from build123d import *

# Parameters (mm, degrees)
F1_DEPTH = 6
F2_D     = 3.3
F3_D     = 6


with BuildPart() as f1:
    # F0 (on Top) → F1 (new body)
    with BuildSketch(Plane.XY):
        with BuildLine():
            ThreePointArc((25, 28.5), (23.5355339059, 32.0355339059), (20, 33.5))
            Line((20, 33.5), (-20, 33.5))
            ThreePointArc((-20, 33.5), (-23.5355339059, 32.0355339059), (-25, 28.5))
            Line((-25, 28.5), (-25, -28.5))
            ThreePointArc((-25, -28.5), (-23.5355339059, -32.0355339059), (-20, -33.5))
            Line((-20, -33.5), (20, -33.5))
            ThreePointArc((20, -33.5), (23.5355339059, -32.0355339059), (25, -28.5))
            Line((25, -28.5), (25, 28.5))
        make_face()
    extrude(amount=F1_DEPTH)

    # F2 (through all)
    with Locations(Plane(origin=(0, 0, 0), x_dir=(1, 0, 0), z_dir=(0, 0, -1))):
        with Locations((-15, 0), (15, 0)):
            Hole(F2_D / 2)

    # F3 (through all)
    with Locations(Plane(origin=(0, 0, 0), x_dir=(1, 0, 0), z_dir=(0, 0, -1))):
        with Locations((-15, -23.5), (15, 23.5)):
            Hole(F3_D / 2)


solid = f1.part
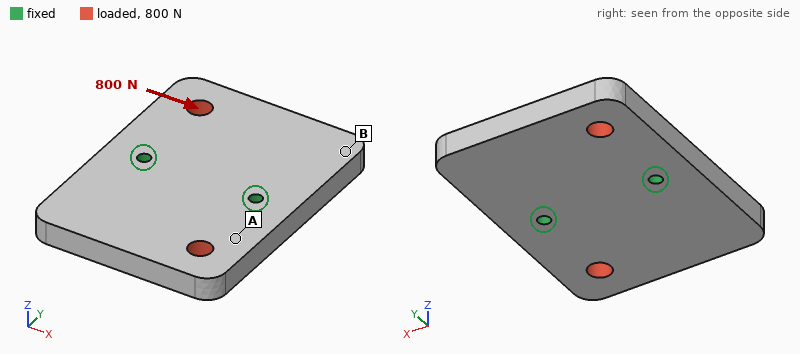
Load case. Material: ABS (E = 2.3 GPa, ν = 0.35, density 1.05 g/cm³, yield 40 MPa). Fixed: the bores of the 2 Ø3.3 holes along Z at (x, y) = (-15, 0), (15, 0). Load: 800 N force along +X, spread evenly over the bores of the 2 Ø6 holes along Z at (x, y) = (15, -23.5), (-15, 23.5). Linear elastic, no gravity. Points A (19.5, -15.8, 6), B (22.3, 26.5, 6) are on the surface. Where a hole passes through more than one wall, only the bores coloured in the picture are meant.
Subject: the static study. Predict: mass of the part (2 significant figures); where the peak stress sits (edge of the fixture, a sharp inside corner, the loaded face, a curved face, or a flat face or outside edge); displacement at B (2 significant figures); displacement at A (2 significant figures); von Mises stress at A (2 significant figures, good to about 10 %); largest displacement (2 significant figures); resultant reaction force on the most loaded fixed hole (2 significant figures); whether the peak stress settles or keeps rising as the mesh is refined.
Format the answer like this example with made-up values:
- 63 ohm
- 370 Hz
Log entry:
- 21 g
- edge of the fixture
- 55 µm
- 51 µm
- 2.5 MPa
- 87 µm
- 400 N
- keeps rising
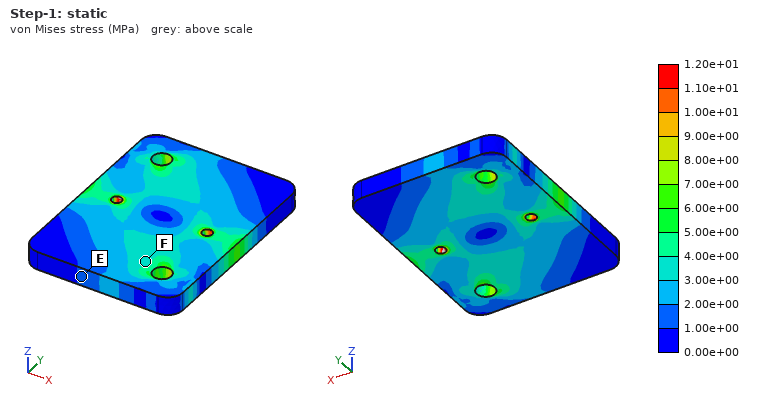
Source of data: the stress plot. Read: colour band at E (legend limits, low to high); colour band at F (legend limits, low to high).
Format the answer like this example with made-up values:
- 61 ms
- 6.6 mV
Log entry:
- 1.00e+00 to 2.00e+00 MPa
- 3.00e+00 to 4.00e+00 MPa
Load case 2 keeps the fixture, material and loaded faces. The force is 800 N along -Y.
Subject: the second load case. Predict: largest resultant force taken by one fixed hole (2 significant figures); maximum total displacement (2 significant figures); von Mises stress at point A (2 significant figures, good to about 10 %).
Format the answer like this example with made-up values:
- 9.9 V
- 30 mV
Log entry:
- 400 N
- 56 µm
- 3.8 MPa
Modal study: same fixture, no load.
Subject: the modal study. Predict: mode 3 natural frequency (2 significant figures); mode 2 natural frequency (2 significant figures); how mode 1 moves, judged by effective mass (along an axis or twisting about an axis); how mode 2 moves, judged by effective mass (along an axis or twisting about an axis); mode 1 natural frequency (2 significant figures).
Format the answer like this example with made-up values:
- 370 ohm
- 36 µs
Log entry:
- 2000 Hz
- 1300 Hz
- twisting about X
- along Z
- 1000 Hz
